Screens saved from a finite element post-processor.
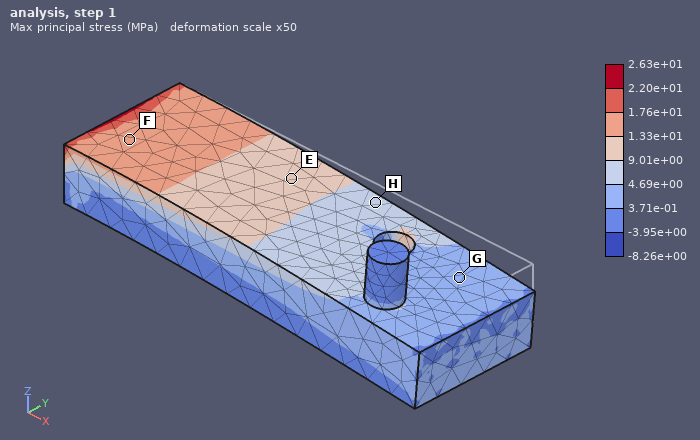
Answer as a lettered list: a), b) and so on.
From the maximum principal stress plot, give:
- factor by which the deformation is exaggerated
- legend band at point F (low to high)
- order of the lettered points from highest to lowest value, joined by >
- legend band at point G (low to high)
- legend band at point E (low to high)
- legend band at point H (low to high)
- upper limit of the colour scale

a) 50
b) 1.33e+01 to 1.76e+01 MPa
c) F > E > H > G
d) 3.71e-01 to 4.69e+00 MPa
e) 9.01e+00 to 1.33e+01 MPa
f) 4.69e+00 to 9.01e+00 MPa
g) 2.63e+01 MPa
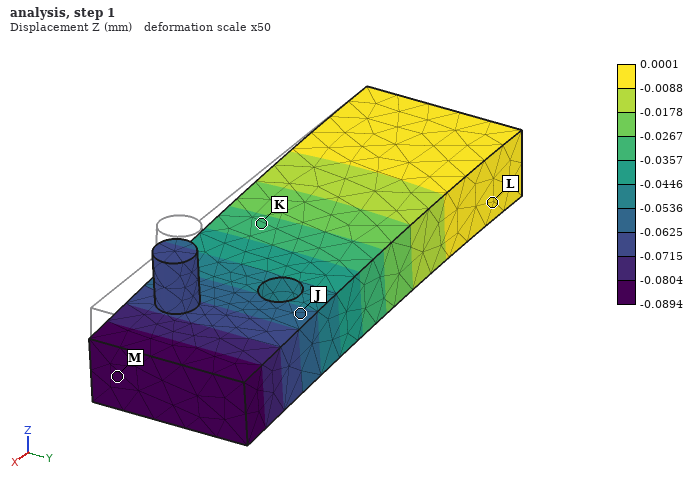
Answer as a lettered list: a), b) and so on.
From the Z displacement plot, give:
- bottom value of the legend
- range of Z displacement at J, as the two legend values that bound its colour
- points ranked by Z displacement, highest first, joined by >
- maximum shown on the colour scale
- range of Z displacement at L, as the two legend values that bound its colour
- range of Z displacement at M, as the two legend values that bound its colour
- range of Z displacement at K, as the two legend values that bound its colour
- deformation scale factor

a) -0.0894 mm
b) -0.0625 to -0.0536 mm
c) L > K > J > M
d) 0.0001 mm
e) -0.0088 to 0.0001 mm
f) -0.0894 to -0.0804 mm
g) -0.0357 to -0.0267 mm
h) 50
